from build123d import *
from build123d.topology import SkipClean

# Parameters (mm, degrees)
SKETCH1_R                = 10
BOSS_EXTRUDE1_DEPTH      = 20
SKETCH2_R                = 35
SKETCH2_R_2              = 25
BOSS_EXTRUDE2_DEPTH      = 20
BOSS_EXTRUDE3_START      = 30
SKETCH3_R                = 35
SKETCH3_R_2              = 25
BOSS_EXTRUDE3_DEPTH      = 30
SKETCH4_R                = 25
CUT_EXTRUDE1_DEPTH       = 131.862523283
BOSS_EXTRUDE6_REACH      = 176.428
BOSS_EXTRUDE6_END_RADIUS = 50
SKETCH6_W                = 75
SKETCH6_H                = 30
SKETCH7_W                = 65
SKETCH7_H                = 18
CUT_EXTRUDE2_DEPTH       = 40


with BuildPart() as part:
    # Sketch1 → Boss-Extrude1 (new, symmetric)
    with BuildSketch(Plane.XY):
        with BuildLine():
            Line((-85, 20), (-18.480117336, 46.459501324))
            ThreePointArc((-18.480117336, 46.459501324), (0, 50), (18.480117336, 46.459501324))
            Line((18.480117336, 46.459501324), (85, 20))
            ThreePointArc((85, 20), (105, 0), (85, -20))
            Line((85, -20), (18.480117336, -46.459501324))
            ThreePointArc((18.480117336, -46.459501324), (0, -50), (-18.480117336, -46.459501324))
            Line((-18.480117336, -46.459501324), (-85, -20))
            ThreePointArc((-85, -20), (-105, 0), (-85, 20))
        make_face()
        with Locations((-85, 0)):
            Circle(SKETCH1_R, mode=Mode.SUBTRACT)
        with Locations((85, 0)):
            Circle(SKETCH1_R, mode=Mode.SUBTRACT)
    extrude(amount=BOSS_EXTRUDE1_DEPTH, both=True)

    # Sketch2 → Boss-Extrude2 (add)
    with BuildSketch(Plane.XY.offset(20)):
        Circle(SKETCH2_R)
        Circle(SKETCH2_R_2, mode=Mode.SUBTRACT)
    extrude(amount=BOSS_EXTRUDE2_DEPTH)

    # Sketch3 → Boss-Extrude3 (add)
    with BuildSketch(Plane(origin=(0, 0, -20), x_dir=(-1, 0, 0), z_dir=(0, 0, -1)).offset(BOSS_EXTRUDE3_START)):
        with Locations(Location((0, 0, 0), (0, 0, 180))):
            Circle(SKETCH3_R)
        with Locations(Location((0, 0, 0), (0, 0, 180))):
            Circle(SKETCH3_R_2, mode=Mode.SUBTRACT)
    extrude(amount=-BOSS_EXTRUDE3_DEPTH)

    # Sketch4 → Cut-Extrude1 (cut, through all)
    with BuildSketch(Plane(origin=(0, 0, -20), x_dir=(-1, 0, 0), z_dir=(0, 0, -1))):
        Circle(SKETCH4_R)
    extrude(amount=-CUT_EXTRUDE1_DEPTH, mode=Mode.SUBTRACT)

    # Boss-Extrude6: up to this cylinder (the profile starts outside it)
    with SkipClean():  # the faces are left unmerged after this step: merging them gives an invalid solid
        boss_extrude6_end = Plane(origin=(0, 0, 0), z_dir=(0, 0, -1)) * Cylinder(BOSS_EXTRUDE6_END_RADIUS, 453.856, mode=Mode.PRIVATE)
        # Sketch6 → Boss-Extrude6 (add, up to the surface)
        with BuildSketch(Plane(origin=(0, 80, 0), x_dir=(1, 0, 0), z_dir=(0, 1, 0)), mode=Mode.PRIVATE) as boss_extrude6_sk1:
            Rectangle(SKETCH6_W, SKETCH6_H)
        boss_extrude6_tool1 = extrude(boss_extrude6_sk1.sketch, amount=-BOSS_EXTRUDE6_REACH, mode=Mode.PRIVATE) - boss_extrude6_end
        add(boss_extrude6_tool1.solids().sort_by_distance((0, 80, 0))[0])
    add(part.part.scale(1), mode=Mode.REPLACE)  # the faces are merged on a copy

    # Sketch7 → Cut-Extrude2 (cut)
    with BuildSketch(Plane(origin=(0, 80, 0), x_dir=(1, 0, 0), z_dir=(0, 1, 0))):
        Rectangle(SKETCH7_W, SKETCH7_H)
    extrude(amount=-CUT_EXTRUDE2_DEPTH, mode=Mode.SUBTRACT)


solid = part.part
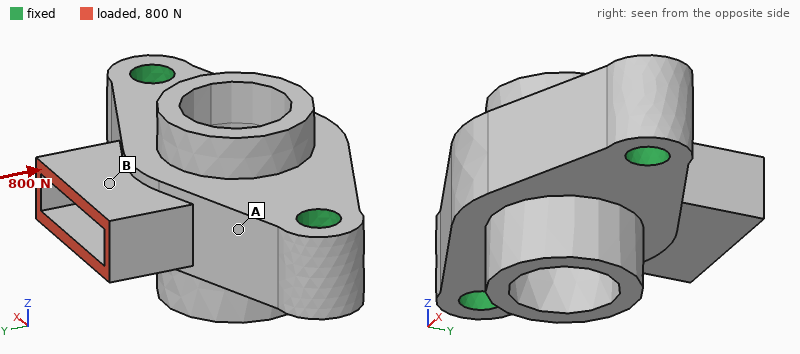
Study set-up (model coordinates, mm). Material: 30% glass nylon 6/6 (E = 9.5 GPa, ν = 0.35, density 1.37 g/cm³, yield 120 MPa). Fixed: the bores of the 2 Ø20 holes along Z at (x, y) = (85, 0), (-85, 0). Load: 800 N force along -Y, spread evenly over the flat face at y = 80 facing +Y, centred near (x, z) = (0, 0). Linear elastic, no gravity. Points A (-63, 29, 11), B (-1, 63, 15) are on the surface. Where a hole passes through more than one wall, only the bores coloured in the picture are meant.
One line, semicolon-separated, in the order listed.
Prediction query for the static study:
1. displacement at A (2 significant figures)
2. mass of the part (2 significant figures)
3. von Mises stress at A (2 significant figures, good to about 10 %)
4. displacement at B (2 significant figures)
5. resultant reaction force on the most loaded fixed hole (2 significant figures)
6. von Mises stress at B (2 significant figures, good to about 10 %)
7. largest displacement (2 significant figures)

1.9 µm; 780 g; 0.20 MPa; 6.5 µm; 420 N; 0.67 MPa; 8.1 µm
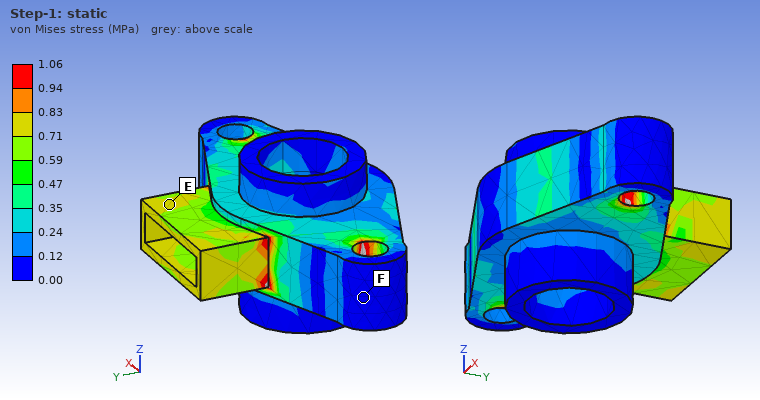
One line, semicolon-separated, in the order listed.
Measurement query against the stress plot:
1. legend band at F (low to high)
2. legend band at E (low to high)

0.00 to 0.12 MPa; 0.71 to 0.83 MPa
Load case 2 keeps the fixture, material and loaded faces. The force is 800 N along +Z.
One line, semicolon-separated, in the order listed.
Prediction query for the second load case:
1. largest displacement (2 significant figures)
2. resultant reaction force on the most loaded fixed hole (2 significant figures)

0.22 mm; 400 N
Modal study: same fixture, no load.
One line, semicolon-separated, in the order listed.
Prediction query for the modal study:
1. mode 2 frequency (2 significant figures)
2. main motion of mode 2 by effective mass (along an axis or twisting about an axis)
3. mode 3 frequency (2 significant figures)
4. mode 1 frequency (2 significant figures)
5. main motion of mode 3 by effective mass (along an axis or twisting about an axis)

2400 Hz; along Z; 3000 Hz; 1800 Hz; along Y
